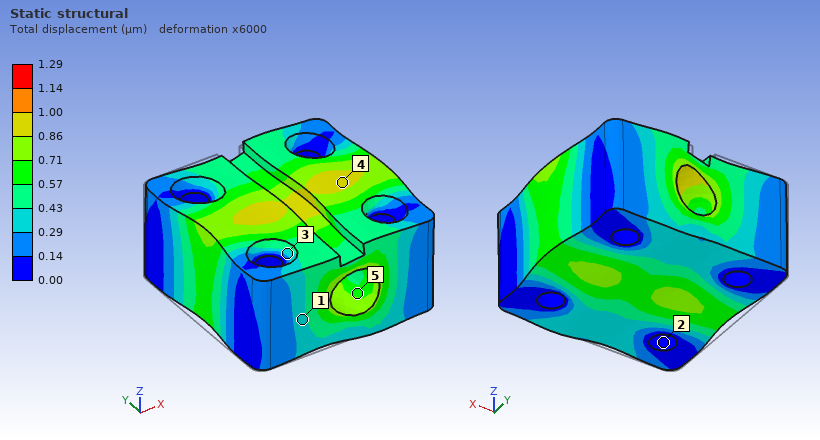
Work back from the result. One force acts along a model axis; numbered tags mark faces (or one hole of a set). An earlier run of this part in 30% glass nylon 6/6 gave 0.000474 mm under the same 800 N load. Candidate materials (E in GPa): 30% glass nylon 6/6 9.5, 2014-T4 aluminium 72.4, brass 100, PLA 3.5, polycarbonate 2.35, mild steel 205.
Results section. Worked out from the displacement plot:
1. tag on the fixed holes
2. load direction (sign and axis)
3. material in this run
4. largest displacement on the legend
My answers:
2
+X
PLA
1.29 µm
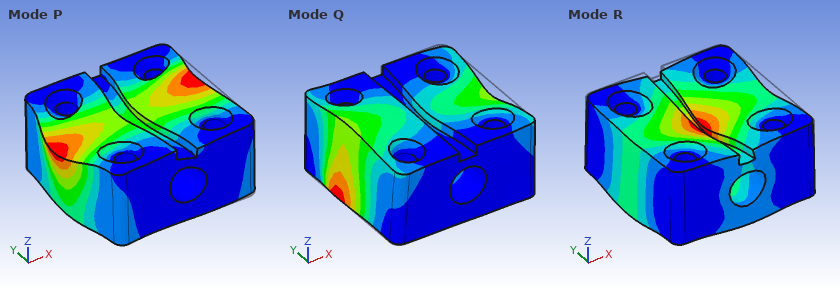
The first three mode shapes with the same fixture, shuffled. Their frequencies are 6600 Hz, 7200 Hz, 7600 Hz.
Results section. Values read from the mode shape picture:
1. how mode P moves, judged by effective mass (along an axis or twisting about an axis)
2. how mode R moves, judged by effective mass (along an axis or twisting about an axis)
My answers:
along X
along Z
